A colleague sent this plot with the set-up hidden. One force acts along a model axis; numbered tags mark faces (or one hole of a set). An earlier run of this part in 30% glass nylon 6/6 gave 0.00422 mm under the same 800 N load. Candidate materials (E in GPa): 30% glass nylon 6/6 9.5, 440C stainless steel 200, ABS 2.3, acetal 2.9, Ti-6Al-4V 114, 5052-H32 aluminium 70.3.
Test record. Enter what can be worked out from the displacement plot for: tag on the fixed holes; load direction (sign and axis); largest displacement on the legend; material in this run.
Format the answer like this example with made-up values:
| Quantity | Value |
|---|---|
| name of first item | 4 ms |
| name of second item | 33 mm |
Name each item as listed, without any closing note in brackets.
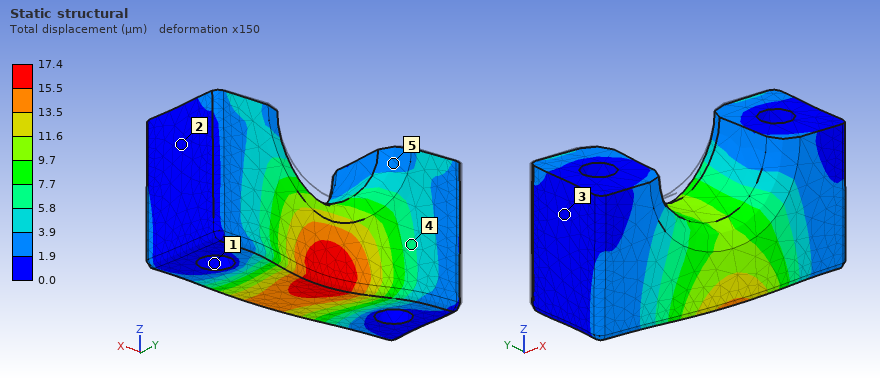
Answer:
| Quantity | Value |
|---|---|
| tag on the fixed holes | 1 |
| load direction | -Y |
| largest displacement on the legend | 17.4 µm |
| material in this run | ABS |
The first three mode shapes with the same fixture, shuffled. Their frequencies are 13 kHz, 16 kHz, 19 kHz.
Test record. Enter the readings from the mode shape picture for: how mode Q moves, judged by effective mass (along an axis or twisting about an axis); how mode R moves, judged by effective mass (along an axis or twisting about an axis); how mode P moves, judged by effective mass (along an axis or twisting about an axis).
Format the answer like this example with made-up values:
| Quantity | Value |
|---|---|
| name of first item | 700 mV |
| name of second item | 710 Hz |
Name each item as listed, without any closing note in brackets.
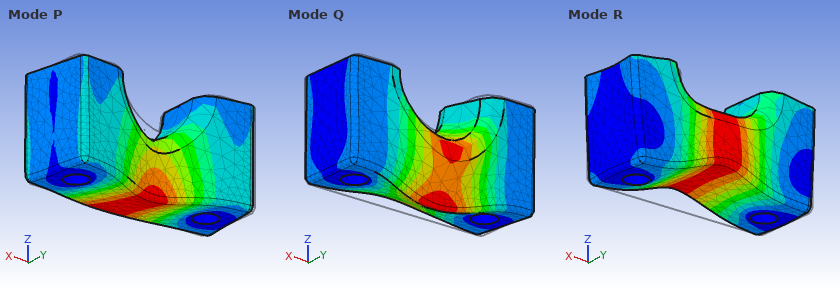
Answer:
| Quantity | Value |
|---|---|
| how mode Q moves, judged by effective mass | twisting about X |
| how mode R moves, judged by effective mass | along Z |
| how mode P moves, judged by effective mass | along Y |
